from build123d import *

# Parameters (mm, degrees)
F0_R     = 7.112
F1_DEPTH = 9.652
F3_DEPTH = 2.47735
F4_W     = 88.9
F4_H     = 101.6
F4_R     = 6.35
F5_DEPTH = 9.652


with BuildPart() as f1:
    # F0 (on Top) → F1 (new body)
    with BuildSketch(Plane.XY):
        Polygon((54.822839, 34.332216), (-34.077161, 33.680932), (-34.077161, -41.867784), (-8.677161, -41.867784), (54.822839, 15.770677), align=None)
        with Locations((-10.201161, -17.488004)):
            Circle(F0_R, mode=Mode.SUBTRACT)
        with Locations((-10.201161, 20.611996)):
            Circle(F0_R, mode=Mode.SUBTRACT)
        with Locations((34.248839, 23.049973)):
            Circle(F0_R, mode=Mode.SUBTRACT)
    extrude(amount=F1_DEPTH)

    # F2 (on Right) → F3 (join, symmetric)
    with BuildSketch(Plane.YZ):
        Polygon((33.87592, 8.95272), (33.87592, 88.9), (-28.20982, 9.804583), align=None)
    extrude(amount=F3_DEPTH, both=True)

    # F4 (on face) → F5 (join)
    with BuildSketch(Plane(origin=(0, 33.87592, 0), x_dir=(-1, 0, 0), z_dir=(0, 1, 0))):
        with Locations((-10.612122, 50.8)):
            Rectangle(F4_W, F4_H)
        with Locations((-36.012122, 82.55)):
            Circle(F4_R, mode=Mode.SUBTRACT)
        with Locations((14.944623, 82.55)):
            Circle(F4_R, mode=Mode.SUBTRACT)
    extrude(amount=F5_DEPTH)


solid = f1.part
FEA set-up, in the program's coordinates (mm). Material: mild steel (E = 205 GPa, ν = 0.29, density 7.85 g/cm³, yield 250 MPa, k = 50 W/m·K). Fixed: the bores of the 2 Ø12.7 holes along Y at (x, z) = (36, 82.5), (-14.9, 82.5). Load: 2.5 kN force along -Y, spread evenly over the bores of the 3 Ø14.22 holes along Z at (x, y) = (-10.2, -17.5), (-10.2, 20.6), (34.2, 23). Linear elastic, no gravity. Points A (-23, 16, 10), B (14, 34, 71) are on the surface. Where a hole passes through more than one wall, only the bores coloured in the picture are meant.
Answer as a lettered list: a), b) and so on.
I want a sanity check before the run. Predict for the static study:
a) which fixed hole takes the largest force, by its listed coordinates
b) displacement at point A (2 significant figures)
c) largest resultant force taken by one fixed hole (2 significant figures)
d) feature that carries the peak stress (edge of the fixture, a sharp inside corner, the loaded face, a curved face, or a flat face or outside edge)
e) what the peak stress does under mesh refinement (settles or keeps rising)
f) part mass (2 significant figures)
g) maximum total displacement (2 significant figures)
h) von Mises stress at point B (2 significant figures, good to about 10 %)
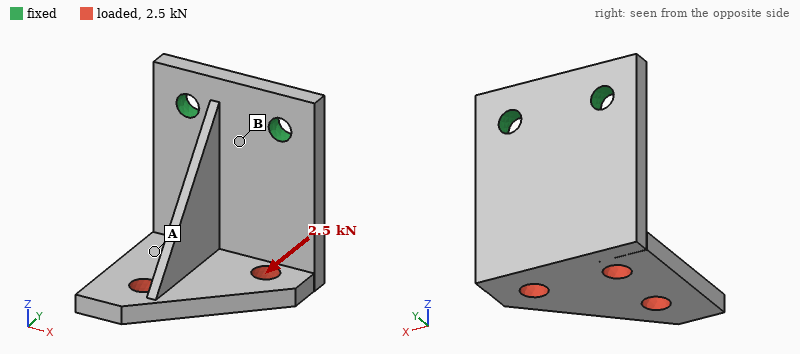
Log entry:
a) (-14.9, 82.5)
b) 0.16 mm
c) 1.4 kN
d) edge of the fixture
e) keeps rising
f) 1.1 kg
g) 0.25 mm
h) 54 MPa
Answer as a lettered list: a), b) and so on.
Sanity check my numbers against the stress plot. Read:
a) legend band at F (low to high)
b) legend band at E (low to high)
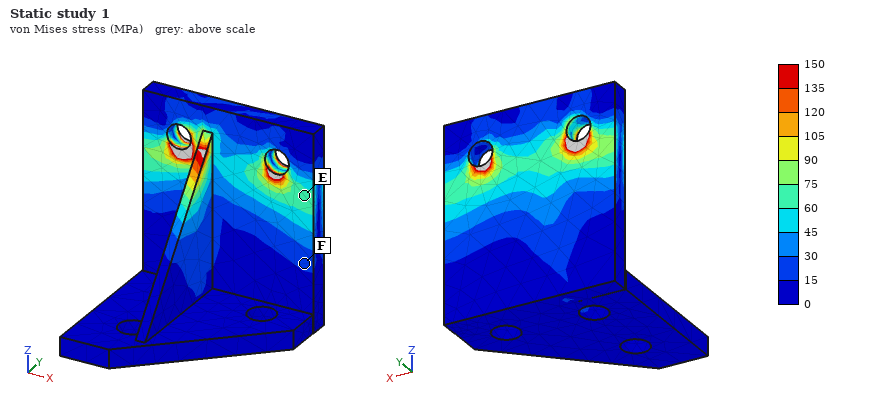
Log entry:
a) 15 to 30 MPa
b) 60 to 75 MPa
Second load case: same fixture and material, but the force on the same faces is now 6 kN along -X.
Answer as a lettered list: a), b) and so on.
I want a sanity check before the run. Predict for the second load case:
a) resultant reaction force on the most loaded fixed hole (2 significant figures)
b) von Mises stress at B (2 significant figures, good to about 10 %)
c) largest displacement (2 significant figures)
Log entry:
a) 8.8 kN
b) 57 MPa
c) 0.40 mm
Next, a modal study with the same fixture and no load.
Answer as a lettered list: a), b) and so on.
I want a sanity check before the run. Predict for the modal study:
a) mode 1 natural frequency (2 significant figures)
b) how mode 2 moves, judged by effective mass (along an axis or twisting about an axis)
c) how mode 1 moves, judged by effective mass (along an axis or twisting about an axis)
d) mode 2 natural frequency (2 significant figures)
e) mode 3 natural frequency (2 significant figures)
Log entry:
a) 770 Hz
b) along X
c) along Y
d) 1100 Hz
e) 2800 Hz
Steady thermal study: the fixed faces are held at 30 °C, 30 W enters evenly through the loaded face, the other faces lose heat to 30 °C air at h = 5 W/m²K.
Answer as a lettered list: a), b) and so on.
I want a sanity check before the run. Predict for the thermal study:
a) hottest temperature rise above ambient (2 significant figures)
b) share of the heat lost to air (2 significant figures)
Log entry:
a) 65 K
b) 19 %
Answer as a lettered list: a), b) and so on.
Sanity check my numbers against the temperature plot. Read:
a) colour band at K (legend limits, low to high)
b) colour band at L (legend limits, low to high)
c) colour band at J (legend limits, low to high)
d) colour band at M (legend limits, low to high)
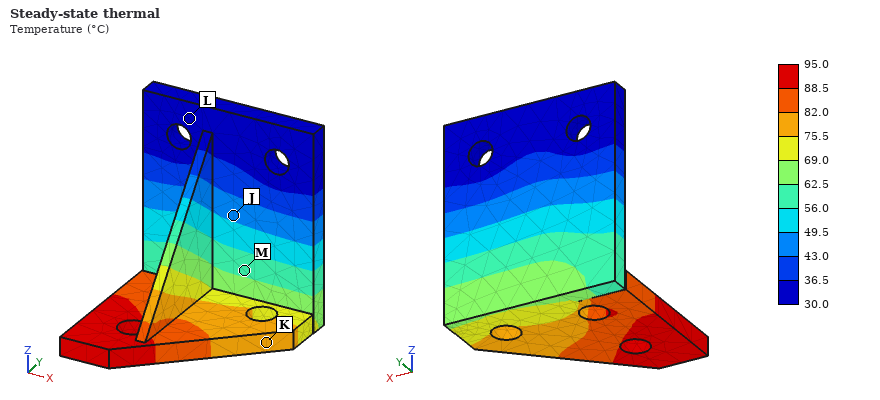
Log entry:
a) 75.5 to 82.0 °C
b) 30.0 to 36.5 °C
c) 43.0 to 49.5 °C
d) 56.0 to 62.5 °C
